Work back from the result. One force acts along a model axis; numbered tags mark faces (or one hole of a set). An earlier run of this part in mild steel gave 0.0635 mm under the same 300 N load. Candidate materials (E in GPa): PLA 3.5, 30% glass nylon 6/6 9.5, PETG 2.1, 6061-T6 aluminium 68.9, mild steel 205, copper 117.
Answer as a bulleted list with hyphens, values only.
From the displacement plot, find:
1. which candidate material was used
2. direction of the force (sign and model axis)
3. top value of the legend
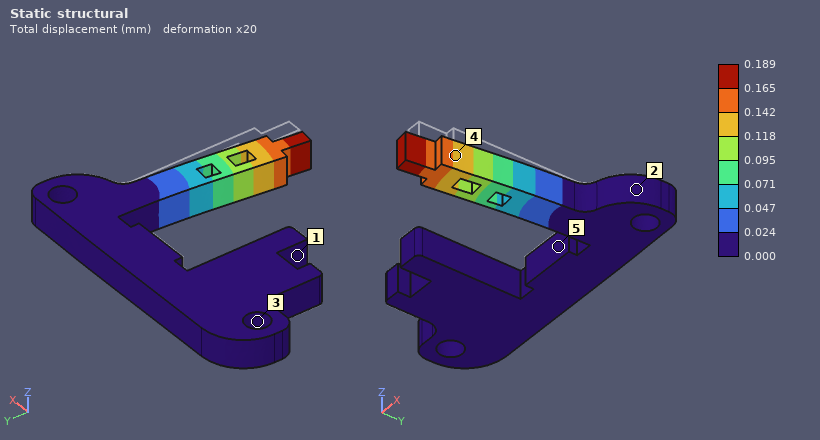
- 6061-T6 aluminium
- -X
- 0.189 mm
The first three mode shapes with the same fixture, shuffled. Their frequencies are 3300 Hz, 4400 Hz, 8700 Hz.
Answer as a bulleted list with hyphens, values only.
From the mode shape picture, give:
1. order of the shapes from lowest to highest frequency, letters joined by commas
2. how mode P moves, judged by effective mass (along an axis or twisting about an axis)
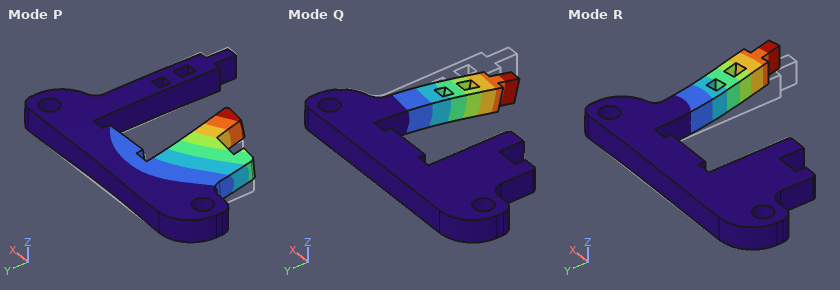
- Q, R, P
- along Z
